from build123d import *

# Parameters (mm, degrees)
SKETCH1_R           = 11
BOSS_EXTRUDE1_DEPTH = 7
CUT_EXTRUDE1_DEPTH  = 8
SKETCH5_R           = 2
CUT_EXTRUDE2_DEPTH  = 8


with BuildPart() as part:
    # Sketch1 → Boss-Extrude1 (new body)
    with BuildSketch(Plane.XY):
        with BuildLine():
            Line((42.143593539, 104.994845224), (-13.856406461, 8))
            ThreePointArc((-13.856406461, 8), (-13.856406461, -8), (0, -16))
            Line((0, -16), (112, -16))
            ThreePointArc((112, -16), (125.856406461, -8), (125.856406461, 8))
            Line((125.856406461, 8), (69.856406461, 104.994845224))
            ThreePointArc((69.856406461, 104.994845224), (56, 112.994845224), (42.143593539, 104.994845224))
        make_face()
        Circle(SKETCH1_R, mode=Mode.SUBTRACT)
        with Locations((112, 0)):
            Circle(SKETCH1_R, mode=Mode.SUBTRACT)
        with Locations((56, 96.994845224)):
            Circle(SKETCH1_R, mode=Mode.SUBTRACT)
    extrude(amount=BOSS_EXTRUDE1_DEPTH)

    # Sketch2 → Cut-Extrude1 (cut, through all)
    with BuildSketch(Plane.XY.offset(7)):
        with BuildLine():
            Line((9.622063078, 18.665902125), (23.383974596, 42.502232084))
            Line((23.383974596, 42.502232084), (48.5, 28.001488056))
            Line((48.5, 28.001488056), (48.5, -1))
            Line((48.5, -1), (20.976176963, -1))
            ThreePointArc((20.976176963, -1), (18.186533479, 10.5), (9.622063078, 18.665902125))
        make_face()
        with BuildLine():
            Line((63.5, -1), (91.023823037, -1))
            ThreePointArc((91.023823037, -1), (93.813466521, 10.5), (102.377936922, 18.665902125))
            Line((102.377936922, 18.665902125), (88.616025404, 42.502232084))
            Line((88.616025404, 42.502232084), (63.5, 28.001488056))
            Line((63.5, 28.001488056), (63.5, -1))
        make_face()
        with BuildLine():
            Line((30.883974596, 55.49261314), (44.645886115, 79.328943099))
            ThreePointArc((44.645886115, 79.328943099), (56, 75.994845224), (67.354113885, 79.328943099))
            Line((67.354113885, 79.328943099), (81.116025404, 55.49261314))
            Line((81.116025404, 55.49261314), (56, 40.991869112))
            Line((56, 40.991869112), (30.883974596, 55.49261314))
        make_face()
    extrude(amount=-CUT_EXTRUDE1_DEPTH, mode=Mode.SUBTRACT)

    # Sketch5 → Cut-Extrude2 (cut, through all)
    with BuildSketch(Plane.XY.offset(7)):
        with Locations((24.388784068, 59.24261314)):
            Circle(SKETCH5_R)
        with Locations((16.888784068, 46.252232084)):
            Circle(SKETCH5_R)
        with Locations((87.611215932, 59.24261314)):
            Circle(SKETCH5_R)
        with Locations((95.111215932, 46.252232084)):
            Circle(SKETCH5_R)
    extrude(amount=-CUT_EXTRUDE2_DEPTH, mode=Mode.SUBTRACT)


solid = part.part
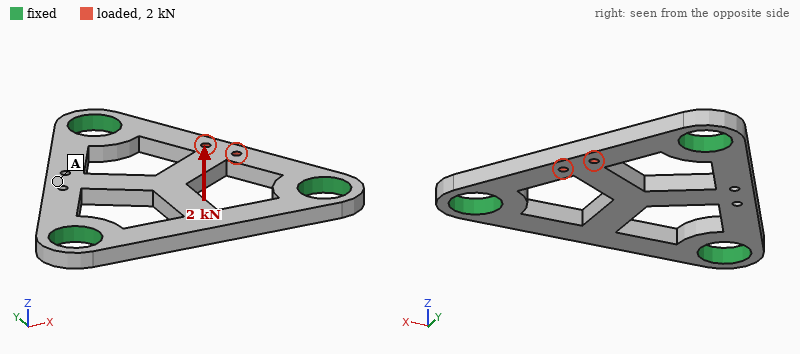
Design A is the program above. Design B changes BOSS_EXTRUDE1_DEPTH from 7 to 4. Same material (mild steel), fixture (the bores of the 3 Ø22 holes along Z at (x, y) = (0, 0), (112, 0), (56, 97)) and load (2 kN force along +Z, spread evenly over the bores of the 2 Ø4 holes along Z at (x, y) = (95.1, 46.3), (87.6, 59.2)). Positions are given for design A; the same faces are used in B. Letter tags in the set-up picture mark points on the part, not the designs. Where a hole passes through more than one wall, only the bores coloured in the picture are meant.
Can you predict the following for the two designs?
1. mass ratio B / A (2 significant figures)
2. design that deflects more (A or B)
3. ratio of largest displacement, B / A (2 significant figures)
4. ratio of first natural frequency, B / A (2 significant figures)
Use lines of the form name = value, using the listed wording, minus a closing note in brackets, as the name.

mass ratio B / A = 0.57
design that deflects more = B
ratio of largest displacement, B / A = 5.0
ratio of first natural frequency, B / A = 0.60
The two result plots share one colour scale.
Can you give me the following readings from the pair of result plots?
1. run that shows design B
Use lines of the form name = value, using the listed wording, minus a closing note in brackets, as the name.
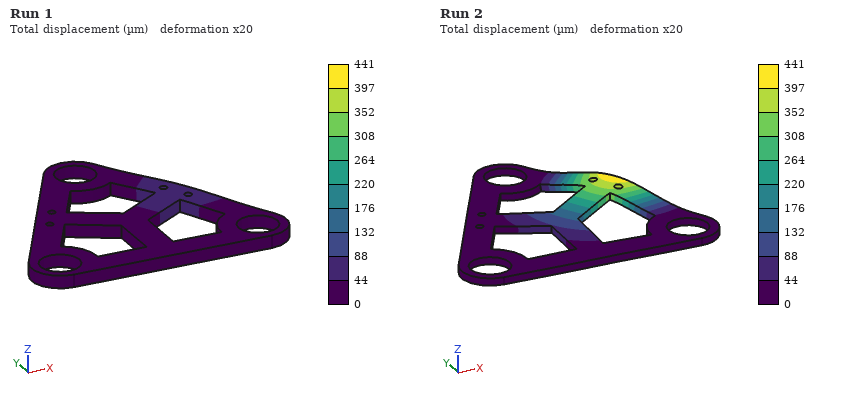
run that shows design B = Run 2
